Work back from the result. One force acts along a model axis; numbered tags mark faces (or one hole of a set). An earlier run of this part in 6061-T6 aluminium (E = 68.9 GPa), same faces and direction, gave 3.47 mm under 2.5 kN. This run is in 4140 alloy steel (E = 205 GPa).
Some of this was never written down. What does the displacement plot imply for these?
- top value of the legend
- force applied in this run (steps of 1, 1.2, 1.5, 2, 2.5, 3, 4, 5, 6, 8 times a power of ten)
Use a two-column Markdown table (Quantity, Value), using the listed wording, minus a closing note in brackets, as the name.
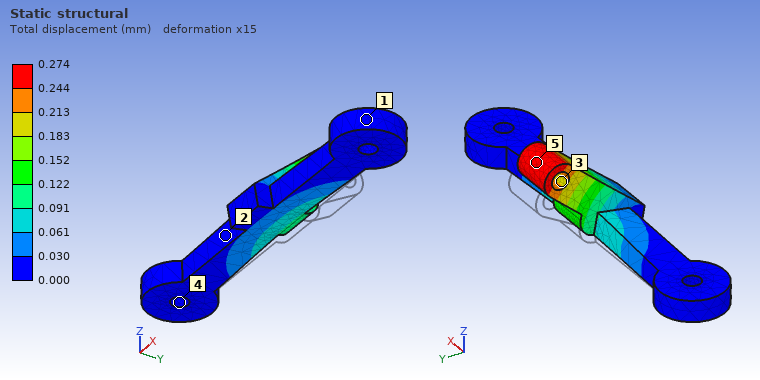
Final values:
| Quantity | Value |
|---|---|
| top value of the legend | 0.274 mm |
| force applied in this run | 600 N |
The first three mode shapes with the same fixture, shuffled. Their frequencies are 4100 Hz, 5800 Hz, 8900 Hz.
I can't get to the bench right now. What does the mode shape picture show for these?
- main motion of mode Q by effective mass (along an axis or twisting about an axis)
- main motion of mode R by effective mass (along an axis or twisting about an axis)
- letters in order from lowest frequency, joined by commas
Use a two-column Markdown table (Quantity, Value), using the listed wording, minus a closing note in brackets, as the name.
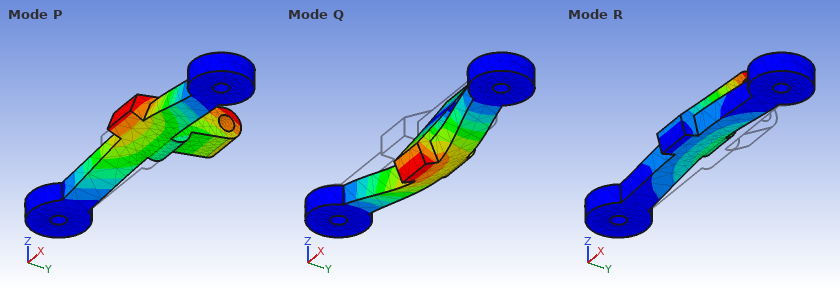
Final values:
| Quantity | Value |
|---|---|
| main motion of mode Q by effective mass | along Y |
| main motion of mode R by effective mass | along Z |
| letters in order from lowest frequency, joined by commas | R, P, Q |
